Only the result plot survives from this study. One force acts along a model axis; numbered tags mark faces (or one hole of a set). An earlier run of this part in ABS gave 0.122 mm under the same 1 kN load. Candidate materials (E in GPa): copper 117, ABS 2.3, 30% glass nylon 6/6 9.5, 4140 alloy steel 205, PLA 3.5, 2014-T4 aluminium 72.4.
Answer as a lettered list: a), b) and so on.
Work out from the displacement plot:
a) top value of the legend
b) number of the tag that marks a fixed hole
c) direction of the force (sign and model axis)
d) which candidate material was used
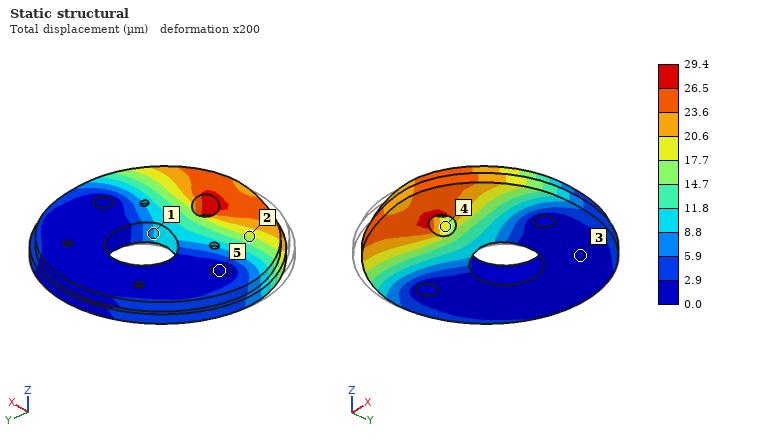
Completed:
a) 29.4 µm
b) 5
c) +X
d) 30% glass nylon 6/6
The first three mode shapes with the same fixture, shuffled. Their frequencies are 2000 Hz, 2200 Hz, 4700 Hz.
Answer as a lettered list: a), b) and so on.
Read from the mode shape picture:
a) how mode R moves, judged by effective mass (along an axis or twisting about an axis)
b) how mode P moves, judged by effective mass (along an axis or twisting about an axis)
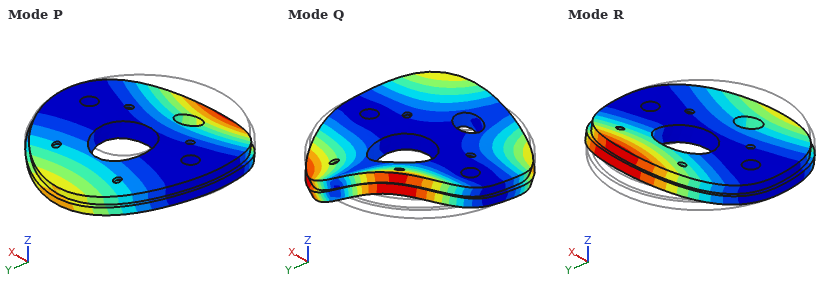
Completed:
a) twisting about X
b) along Z
